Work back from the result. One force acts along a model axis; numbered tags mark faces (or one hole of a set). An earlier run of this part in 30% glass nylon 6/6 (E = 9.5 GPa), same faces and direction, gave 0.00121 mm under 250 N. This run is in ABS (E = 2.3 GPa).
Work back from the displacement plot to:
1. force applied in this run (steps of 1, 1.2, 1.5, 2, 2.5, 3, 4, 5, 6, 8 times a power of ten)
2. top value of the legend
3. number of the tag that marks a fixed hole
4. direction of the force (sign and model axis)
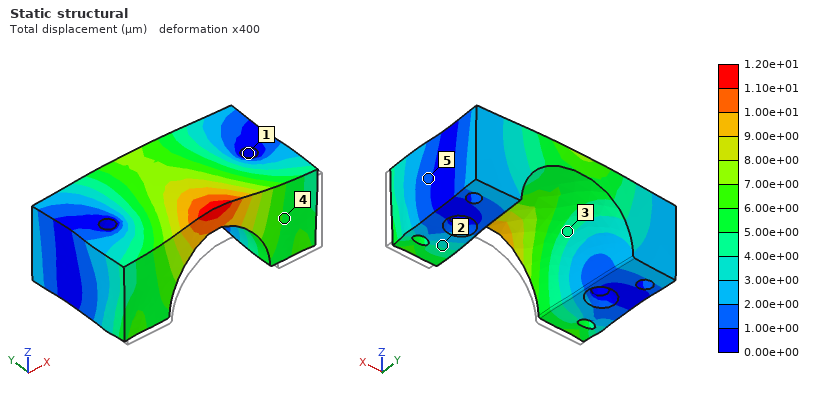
600 N
1.20e+01 µm
1
+Y
